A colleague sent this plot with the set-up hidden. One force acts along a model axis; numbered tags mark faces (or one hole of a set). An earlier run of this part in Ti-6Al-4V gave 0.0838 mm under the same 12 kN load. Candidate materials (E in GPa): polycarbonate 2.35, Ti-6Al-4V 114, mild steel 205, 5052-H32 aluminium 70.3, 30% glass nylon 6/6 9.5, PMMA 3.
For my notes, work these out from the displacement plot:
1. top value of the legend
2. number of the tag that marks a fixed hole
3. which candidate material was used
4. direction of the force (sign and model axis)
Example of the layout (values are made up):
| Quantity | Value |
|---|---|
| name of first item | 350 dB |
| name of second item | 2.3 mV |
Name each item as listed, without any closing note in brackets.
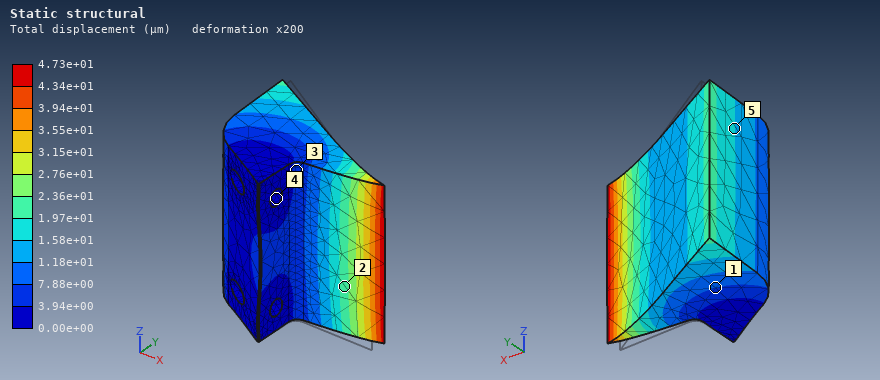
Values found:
| Quantity | Value |
|---|---|
| top value of the legend | 4.73e+01 µm |
| number of the tag that marks a fixed hole | 4 |
| which candidate material was used | mild steel |
| direction of the force | +Y |
